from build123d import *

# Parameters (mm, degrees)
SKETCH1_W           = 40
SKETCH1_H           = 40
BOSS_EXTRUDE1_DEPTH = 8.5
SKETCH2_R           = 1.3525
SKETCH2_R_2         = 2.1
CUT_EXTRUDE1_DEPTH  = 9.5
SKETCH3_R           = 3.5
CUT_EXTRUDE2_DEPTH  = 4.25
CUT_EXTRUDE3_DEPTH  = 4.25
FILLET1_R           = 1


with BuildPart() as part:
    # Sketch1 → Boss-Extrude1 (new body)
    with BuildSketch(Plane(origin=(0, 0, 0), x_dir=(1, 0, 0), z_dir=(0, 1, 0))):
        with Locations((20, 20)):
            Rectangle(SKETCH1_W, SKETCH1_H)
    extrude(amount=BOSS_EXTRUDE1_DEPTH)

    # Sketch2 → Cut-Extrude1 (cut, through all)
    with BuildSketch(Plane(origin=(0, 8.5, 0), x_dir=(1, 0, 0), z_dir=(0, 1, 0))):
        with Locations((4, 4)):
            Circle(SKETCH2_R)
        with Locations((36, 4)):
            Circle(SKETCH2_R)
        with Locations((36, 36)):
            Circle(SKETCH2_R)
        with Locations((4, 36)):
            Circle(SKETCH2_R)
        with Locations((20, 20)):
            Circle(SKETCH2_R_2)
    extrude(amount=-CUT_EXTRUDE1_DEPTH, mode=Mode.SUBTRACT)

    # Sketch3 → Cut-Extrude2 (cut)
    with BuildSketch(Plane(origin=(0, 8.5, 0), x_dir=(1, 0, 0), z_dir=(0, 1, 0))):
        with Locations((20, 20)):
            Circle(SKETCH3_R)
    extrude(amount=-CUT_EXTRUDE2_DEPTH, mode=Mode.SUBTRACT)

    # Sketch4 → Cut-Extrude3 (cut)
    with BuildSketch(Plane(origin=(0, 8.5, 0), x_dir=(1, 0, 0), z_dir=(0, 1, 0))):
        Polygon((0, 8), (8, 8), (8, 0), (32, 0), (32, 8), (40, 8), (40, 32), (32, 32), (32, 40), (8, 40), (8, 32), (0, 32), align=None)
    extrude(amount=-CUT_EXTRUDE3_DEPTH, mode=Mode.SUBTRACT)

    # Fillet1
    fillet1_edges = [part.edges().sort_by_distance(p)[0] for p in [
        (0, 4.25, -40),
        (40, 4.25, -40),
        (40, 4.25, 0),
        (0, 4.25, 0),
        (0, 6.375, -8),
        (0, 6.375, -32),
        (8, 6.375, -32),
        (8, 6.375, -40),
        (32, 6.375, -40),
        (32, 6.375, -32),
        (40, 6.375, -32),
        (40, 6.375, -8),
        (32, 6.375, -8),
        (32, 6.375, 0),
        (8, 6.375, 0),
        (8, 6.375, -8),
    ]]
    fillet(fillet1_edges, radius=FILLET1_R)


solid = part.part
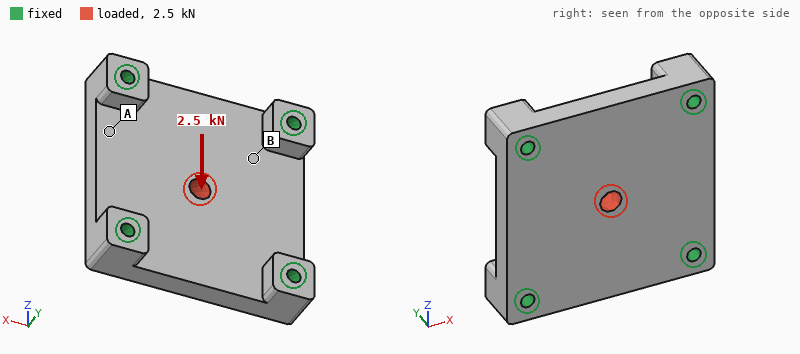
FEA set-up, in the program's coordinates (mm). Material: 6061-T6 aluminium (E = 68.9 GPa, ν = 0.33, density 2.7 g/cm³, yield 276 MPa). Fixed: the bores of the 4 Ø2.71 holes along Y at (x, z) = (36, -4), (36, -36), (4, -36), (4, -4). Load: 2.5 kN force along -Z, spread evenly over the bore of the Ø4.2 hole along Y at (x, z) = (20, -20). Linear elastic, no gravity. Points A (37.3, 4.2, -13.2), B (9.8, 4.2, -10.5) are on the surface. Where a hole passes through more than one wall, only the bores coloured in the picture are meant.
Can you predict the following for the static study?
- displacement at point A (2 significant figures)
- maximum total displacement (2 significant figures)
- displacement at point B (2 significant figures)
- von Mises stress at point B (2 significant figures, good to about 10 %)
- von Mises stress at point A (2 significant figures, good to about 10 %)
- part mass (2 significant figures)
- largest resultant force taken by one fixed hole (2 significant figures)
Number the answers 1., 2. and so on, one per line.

1. 1.2 µm
2. 7.8 µm
3. 2.5 µm
4. 19 MPa
5. 7.6 MPa
6. 21 g
7. 710 N
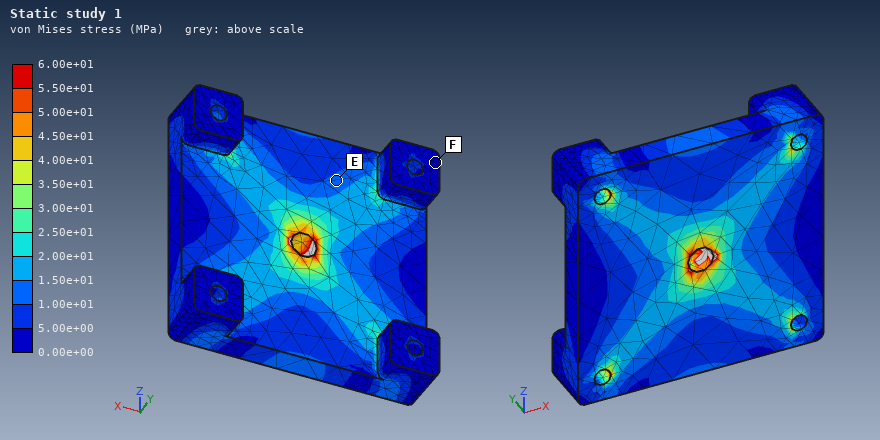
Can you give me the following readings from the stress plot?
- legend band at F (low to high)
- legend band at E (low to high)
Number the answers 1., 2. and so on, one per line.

1. 0.00e+00 to 5.00e+00 MPa
2. 1.00e+01 to 1.50e+01 MPa
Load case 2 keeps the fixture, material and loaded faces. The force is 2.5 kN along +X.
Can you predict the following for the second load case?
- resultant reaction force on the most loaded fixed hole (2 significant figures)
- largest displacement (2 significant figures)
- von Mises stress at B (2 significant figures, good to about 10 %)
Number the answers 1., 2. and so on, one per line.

1. 710 N
2. 7.9 µm
3. 19 MPa
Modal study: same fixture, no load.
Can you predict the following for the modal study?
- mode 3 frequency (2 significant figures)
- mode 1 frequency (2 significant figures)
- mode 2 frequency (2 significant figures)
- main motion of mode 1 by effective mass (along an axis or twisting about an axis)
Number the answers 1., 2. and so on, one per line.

1. 25 kHz
2. 16 kHz
3. 25 kHz
4. along Y
